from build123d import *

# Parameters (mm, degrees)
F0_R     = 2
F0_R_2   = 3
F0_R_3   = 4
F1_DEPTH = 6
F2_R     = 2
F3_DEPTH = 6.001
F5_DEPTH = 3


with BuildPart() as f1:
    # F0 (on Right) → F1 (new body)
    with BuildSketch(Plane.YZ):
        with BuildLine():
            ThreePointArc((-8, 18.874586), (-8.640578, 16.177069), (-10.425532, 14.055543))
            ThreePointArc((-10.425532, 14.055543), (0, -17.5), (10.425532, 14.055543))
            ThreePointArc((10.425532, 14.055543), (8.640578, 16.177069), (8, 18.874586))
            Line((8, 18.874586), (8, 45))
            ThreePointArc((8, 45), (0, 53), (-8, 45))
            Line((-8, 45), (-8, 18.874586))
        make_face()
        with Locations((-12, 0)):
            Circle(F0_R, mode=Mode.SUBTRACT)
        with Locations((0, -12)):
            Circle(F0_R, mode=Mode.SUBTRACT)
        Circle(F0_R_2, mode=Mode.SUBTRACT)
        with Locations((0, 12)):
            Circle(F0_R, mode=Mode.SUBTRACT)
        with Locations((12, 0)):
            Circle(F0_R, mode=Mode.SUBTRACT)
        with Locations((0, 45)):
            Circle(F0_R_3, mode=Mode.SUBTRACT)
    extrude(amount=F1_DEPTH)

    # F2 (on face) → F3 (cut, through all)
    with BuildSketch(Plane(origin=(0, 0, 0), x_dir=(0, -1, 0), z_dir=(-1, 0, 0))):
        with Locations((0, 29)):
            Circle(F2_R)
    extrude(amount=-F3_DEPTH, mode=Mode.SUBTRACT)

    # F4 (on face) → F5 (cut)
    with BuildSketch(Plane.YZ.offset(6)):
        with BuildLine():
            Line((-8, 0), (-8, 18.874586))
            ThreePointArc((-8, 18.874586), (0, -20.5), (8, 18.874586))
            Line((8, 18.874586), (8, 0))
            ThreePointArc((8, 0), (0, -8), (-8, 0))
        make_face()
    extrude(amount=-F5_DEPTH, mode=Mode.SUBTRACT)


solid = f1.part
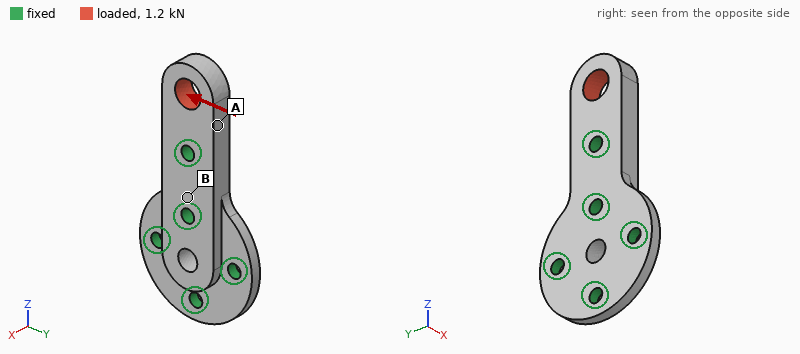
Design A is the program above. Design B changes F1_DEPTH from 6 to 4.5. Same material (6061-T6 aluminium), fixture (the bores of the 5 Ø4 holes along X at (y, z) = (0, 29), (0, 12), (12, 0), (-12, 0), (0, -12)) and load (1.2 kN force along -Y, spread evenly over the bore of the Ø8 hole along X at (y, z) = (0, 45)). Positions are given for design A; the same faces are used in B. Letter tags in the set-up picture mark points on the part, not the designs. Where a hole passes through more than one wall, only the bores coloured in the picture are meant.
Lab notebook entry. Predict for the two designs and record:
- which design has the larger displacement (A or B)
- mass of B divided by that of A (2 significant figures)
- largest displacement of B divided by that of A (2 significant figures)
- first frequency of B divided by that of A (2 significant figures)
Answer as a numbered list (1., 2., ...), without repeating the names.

1. B
2. 0.81
3. 1.3
4. 0.79
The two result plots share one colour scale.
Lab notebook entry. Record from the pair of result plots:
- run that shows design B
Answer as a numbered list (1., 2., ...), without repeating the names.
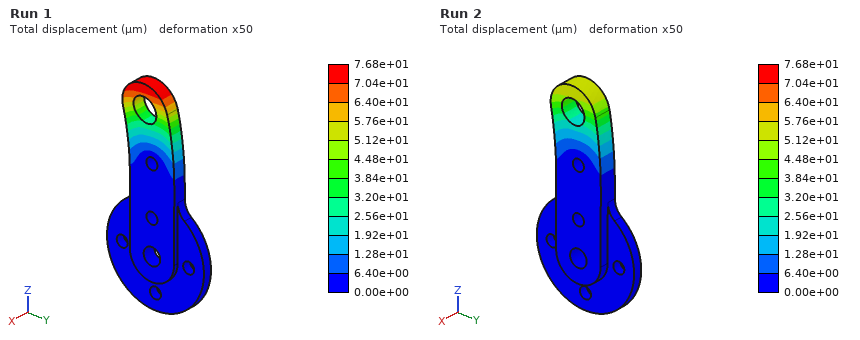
1. Run 1
